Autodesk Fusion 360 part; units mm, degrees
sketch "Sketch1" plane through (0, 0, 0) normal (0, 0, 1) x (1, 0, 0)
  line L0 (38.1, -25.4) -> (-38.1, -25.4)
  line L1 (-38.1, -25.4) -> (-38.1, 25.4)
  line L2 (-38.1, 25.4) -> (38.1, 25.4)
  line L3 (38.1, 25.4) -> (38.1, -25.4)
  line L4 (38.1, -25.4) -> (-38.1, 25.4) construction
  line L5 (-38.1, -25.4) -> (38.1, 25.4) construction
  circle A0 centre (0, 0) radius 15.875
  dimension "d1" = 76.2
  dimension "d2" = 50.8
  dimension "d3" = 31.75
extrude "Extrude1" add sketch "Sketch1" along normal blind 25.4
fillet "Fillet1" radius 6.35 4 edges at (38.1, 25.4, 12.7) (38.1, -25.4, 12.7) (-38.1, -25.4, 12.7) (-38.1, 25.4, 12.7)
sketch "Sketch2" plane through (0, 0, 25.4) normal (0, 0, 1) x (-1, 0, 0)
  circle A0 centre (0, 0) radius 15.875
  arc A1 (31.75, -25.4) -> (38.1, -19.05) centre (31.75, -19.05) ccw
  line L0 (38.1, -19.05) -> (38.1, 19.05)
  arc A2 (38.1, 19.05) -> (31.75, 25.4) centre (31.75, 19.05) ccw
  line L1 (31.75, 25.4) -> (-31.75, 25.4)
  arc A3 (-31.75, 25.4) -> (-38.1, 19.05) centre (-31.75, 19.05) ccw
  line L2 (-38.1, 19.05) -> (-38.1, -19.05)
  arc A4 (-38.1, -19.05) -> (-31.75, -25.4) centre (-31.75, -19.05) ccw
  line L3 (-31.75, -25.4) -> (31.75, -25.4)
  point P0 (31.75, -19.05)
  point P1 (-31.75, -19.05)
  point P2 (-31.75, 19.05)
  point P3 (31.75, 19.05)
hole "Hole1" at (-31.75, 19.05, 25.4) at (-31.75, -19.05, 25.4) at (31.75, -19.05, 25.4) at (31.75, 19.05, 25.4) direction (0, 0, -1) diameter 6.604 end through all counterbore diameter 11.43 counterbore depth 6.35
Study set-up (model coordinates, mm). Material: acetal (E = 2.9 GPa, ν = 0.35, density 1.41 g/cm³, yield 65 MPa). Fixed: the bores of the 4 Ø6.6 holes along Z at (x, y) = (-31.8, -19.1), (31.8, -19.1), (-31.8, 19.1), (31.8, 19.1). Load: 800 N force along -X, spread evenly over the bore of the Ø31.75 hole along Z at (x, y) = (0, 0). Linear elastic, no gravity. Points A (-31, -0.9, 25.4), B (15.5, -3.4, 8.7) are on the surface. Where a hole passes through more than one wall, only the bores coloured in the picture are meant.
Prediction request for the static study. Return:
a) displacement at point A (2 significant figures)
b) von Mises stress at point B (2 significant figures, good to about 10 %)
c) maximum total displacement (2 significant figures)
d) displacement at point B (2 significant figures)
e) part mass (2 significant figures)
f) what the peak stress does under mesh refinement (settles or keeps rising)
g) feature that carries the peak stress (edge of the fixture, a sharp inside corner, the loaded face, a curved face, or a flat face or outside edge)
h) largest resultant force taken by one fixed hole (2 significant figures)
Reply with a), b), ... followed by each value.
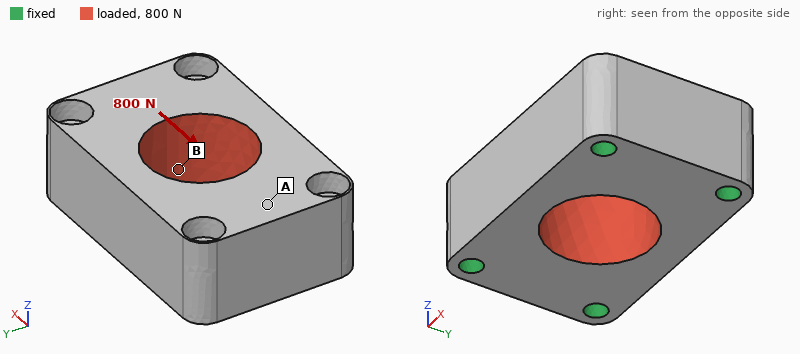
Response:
a) 4.5 µm
b) 0.31 MPa
c) 5.7 µm
d) 4.1 µm
e) 100 g
f) keeps rising
g) edge of the fixture
h) 210 N
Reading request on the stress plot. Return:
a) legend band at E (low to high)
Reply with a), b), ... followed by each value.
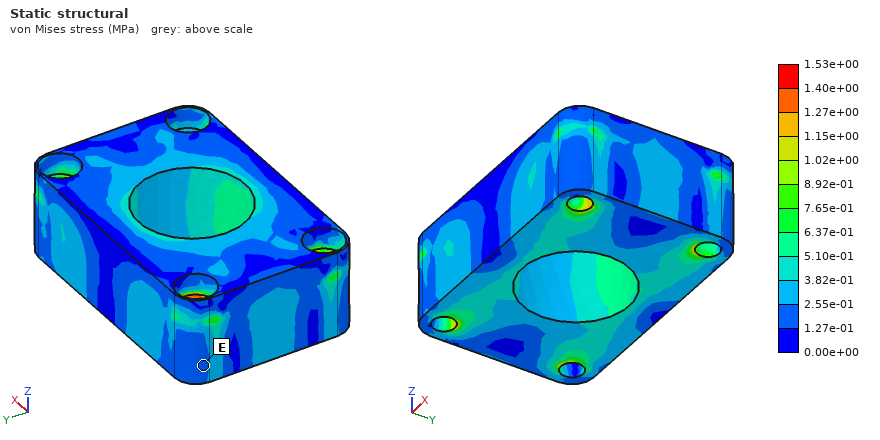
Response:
a) 1.27e-01 to 2.55e-01 MPa
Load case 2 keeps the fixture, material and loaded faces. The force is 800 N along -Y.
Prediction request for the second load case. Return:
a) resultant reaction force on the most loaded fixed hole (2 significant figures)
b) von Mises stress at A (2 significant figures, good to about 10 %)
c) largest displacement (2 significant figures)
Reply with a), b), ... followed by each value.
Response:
a) 230 N
b) 0.43 MPa
c) 15 µm
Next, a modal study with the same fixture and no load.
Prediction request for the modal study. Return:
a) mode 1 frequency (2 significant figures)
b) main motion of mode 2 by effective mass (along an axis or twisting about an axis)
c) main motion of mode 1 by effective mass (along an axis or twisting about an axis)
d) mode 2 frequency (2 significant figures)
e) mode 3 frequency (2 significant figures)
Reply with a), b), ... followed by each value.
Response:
a) 4800 Hz
b) twisting about X
c) along Z
d) 5800 Hz
e) 6300 Hz
